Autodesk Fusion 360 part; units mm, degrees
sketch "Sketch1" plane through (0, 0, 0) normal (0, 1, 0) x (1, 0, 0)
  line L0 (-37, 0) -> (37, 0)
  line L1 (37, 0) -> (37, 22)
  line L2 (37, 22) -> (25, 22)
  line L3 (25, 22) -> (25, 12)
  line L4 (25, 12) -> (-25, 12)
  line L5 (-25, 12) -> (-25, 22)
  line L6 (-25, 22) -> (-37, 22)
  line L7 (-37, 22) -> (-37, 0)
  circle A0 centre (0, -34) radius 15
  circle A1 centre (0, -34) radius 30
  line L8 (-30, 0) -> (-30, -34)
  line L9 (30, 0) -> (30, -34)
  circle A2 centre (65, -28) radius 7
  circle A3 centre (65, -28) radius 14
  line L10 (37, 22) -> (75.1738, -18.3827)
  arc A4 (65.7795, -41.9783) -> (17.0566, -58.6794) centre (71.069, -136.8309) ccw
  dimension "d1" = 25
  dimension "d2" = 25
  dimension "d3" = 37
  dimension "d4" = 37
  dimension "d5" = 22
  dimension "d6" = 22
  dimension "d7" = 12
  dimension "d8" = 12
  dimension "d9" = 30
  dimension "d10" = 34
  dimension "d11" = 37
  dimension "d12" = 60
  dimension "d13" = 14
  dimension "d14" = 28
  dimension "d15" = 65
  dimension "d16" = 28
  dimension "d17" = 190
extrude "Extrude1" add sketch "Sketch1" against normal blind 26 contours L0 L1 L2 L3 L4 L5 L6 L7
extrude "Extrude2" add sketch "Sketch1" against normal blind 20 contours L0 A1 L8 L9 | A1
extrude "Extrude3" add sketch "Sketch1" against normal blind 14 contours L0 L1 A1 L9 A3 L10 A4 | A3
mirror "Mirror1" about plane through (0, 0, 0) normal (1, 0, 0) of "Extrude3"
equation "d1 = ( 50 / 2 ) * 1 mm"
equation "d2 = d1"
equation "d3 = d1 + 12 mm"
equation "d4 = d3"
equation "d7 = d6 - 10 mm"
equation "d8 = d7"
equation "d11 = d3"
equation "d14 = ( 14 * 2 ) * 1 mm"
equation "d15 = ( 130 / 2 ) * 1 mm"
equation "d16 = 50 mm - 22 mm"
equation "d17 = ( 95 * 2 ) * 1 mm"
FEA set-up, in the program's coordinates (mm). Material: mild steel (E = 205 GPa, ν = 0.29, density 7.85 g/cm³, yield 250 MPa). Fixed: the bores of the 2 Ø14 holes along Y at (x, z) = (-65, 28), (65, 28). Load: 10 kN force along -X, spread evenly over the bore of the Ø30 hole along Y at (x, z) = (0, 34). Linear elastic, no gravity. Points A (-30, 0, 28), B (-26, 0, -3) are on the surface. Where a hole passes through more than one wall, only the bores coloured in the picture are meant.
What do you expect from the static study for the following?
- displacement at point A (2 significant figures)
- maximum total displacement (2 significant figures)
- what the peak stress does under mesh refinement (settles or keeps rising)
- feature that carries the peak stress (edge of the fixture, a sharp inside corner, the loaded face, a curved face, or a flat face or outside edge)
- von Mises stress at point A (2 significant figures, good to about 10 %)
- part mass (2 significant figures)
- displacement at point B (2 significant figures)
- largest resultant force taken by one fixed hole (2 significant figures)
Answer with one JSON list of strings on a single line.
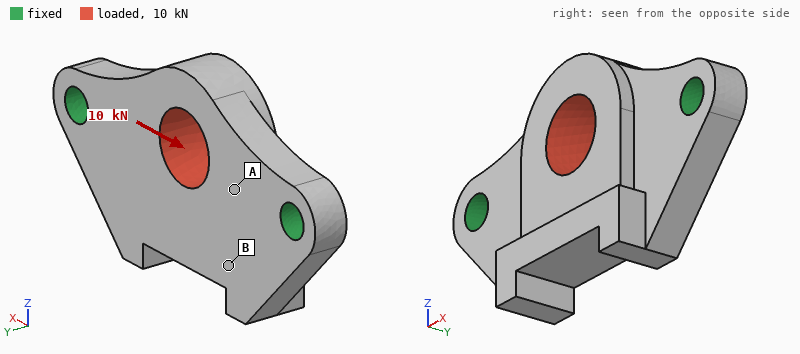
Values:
["1.5 µm", "3.4 µm", "keeps rising", "edge of the fixture", "5.7 MPa", "1.1 kg", "1.3 µm", "5.0 kN"]
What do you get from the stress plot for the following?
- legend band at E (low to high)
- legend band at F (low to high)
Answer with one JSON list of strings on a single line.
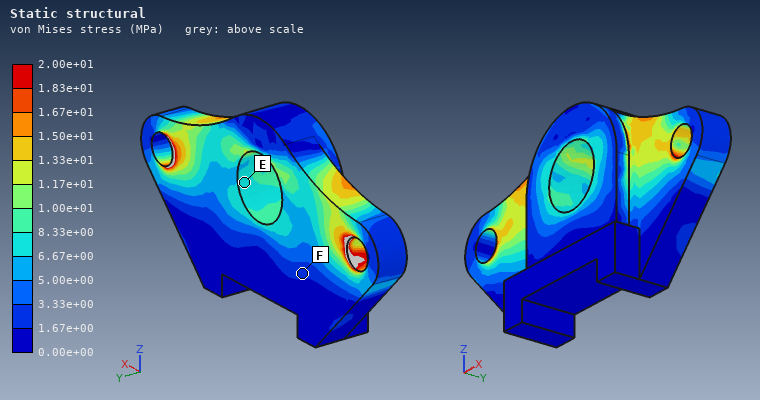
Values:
["6.67e+00 to 8.33e+00 MPa", "1.67e+00 to 3.33e+00 MPa"]
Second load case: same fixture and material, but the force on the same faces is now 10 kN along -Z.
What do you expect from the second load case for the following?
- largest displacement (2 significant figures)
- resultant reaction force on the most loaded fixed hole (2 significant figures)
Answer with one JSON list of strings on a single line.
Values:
["13 µm", "5.2 kN"]
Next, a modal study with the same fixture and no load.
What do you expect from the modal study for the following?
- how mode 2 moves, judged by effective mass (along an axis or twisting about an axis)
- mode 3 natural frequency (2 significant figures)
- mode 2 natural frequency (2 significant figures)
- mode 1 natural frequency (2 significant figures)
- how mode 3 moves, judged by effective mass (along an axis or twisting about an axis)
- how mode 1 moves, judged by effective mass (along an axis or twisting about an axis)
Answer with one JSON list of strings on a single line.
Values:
["along Y", "7100 Hz", "4100 Hz", "2900 Hz", "twisting about Z", "along Y"]
